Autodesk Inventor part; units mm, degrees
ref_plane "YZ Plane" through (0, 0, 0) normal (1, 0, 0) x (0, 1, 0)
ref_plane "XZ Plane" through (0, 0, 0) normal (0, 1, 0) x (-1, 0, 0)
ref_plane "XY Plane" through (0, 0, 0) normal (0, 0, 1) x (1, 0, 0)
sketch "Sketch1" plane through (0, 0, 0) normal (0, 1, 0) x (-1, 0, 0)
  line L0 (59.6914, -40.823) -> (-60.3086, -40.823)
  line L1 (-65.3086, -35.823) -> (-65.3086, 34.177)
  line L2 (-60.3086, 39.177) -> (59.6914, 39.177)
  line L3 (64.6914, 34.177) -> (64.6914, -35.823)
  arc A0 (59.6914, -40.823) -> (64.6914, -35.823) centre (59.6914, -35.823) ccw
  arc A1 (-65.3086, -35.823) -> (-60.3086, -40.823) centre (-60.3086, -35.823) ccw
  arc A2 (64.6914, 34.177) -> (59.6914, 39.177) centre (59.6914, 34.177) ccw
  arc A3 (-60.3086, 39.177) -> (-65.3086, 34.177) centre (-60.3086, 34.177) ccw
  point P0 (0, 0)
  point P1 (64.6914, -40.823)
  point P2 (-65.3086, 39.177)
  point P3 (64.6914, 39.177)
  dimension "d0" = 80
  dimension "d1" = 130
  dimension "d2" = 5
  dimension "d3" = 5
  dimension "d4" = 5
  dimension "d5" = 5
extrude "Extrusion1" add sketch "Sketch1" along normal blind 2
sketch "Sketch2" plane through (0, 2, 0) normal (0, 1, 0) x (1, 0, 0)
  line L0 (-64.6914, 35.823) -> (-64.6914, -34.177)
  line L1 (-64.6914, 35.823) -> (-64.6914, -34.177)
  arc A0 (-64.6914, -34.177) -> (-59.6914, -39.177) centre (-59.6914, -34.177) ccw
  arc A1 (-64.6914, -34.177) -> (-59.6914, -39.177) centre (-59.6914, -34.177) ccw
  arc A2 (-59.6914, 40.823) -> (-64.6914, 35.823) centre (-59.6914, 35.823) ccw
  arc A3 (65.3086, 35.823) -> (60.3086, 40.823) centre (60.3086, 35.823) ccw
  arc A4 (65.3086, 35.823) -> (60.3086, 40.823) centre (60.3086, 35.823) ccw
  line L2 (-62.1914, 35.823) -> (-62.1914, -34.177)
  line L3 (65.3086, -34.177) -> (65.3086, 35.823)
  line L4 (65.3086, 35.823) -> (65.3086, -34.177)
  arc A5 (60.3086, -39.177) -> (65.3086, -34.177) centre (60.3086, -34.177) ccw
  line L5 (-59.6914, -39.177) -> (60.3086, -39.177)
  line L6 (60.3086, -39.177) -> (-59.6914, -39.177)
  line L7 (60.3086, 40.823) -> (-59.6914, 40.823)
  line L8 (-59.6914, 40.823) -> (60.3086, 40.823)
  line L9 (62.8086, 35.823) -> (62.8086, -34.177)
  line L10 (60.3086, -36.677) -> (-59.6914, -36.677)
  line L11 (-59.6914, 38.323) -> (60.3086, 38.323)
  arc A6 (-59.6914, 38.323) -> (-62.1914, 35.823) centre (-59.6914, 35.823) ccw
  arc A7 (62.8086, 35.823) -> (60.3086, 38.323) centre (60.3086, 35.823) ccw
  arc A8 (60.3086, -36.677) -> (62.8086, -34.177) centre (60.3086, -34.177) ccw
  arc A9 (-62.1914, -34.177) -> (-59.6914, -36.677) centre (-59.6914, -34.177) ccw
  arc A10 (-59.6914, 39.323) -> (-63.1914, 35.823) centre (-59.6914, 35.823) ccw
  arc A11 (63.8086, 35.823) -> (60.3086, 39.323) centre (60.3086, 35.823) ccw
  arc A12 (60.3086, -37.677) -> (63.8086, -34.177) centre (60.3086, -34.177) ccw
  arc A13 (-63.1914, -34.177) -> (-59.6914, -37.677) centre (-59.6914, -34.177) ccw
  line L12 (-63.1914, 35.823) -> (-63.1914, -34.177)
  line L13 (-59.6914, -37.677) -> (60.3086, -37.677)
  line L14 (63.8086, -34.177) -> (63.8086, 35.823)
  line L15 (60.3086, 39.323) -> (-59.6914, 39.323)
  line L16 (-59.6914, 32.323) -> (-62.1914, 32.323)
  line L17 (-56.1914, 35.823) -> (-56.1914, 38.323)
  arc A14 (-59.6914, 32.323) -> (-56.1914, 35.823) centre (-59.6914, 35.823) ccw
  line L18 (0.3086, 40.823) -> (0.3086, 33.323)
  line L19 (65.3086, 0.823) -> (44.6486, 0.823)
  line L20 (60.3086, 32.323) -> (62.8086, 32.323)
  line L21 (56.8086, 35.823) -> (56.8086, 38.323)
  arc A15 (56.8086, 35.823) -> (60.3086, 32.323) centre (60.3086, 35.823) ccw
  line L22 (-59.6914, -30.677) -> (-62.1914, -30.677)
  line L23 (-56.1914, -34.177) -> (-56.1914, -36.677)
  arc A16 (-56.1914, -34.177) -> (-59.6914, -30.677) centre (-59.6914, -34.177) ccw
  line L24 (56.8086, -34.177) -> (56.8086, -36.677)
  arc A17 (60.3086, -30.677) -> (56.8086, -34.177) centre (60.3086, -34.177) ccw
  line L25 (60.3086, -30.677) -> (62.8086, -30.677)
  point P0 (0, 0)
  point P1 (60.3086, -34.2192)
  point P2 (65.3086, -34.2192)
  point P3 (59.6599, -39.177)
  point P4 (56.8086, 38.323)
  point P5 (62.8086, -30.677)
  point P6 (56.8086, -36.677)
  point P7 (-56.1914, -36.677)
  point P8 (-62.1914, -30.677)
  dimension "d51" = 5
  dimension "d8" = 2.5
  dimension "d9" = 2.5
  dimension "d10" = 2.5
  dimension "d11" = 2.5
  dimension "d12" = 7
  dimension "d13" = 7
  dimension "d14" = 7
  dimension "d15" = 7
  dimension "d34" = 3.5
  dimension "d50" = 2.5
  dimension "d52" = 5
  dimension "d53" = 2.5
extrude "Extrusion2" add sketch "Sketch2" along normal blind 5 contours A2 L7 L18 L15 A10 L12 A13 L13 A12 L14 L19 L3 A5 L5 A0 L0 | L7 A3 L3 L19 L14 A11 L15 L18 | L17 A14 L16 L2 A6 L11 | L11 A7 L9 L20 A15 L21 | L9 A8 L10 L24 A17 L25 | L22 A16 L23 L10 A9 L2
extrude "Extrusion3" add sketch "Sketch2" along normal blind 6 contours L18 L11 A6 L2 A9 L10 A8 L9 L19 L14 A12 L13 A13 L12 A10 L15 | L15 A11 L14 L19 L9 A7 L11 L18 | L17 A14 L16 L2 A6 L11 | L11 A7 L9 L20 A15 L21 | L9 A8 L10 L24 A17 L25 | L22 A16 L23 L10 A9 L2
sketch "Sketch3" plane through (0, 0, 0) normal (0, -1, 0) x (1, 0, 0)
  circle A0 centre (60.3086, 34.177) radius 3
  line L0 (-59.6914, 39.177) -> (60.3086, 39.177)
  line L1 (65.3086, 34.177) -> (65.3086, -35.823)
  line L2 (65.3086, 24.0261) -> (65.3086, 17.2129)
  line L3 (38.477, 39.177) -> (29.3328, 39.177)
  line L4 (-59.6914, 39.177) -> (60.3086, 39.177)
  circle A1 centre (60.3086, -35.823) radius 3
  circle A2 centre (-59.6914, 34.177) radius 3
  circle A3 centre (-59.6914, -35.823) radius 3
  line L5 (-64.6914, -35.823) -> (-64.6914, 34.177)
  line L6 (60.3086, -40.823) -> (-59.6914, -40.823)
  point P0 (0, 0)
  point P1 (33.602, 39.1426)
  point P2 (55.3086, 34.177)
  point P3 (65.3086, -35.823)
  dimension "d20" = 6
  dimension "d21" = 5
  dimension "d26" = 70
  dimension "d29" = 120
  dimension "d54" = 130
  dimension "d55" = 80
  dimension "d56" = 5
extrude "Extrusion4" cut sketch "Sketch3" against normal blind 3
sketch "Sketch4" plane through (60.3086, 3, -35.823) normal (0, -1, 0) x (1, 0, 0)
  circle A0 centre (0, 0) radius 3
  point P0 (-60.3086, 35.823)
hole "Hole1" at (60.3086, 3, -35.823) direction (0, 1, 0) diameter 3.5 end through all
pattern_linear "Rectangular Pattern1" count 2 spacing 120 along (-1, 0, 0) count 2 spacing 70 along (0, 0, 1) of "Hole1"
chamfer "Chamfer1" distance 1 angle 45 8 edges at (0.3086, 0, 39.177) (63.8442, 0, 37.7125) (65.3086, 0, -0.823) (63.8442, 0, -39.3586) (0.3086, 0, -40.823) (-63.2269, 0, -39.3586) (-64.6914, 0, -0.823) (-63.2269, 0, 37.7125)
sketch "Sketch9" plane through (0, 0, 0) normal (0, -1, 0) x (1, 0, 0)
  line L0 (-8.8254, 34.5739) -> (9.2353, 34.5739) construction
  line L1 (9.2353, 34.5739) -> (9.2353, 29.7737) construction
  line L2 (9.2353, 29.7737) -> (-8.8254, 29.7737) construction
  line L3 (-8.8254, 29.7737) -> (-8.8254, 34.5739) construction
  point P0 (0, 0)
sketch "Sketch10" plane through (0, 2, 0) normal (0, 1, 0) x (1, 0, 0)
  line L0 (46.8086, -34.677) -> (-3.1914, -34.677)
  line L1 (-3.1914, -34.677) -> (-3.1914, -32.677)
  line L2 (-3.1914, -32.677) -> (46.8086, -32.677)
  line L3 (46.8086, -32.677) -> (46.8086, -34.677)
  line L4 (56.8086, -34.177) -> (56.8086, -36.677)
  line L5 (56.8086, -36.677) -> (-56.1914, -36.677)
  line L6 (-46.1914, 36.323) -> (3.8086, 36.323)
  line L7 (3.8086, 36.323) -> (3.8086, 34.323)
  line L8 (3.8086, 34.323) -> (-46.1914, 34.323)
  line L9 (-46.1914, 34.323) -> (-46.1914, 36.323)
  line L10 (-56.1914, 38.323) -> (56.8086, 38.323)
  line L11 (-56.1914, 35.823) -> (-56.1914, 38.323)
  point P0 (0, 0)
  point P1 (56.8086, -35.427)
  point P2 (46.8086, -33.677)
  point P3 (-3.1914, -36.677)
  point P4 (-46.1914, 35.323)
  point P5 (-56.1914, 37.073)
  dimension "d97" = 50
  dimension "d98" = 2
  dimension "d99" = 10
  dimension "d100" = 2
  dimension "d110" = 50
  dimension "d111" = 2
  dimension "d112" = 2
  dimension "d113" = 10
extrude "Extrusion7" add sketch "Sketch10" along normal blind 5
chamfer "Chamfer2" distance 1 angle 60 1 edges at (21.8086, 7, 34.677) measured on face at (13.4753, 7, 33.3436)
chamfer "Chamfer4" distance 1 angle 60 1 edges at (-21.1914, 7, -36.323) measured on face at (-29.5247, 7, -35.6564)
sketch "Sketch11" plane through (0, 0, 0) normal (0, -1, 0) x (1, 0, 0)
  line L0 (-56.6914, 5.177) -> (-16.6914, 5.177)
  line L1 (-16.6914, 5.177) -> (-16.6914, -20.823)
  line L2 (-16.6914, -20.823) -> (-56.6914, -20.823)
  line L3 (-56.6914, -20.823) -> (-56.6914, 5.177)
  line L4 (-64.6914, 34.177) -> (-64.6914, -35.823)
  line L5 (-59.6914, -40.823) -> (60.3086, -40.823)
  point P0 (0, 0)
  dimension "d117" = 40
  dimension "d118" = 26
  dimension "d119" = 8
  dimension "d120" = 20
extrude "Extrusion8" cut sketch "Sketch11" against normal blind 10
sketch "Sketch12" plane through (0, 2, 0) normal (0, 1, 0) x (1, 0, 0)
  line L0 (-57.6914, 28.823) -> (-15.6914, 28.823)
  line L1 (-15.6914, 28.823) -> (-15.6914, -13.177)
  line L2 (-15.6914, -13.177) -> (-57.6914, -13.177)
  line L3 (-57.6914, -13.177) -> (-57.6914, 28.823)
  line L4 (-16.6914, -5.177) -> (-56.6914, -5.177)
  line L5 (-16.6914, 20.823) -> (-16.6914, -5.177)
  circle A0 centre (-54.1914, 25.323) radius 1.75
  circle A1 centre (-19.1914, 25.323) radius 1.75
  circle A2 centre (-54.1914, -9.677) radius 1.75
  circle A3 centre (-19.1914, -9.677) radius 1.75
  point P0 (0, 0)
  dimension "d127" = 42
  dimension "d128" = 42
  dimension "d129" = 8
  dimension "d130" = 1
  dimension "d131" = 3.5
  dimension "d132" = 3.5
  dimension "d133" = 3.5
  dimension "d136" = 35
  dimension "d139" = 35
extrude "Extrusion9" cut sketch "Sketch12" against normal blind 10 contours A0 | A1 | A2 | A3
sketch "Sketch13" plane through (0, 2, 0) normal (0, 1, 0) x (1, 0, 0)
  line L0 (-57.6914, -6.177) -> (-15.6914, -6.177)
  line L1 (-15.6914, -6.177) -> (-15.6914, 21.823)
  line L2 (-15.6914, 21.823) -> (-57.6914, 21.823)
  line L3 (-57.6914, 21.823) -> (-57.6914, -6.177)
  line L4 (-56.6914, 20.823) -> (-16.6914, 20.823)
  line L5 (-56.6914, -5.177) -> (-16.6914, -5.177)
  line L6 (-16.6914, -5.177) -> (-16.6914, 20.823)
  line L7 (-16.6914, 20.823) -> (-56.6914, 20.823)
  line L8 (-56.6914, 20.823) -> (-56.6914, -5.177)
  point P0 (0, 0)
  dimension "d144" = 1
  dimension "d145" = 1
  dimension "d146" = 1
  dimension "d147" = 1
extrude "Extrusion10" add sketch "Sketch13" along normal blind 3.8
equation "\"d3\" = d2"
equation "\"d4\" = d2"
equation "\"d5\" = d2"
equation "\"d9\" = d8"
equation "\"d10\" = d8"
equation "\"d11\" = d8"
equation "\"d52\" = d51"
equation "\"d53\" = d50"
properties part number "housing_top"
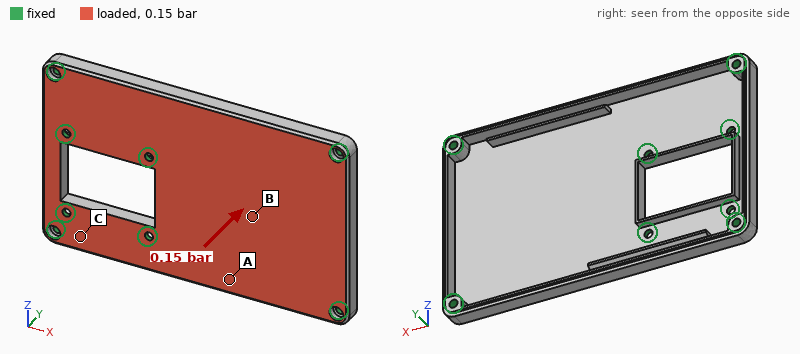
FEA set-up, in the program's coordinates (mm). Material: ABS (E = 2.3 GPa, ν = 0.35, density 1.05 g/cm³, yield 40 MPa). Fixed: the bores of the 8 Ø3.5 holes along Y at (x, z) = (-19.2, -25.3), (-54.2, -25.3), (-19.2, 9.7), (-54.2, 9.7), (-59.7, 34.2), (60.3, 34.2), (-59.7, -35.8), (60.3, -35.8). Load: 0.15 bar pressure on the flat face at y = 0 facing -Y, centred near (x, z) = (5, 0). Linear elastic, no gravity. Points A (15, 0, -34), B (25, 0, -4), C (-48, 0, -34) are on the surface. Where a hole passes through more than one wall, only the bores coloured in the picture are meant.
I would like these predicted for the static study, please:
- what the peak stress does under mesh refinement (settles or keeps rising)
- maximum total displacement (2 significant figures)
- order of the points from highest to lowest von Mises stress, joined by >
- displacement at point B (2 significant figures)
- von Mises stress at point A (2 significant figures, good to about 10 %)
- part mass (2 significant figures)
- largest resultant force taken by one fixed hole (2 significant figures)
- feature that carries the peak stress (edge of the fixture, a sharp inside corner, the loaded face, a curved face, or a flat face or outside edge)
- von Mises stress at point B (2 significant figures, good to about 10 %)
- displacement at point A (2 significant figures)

keeps rising
0.92 mm
B > A > C
0.92 mm
2.7 MPa
27 g
43 N
edge of the fixture
5.2 MPa
0.32 mm
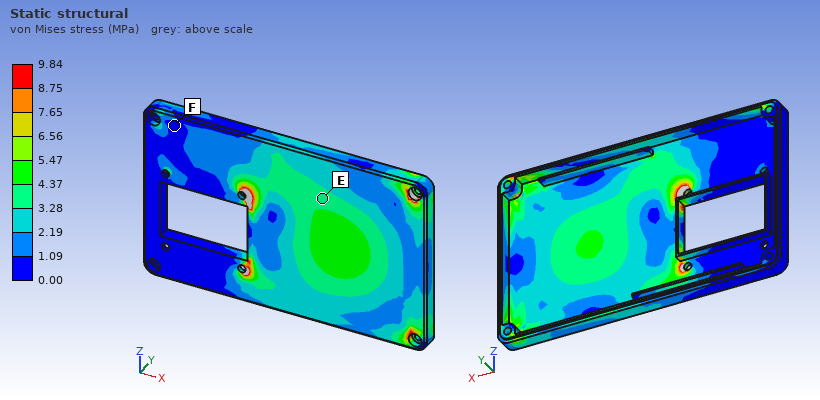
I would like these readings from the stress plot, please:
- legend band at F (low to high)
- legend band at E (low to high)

0.00 to 1.09 MPa
3.28 to 4.37 MPa
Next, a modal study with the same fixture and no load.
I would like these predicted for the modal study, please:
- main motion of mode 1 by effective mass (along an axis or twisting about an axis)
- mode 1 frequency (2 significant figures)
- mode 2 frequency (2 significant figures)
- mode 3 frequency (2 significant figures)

along Y
550 Hz
770 Hz
1000 Hz
